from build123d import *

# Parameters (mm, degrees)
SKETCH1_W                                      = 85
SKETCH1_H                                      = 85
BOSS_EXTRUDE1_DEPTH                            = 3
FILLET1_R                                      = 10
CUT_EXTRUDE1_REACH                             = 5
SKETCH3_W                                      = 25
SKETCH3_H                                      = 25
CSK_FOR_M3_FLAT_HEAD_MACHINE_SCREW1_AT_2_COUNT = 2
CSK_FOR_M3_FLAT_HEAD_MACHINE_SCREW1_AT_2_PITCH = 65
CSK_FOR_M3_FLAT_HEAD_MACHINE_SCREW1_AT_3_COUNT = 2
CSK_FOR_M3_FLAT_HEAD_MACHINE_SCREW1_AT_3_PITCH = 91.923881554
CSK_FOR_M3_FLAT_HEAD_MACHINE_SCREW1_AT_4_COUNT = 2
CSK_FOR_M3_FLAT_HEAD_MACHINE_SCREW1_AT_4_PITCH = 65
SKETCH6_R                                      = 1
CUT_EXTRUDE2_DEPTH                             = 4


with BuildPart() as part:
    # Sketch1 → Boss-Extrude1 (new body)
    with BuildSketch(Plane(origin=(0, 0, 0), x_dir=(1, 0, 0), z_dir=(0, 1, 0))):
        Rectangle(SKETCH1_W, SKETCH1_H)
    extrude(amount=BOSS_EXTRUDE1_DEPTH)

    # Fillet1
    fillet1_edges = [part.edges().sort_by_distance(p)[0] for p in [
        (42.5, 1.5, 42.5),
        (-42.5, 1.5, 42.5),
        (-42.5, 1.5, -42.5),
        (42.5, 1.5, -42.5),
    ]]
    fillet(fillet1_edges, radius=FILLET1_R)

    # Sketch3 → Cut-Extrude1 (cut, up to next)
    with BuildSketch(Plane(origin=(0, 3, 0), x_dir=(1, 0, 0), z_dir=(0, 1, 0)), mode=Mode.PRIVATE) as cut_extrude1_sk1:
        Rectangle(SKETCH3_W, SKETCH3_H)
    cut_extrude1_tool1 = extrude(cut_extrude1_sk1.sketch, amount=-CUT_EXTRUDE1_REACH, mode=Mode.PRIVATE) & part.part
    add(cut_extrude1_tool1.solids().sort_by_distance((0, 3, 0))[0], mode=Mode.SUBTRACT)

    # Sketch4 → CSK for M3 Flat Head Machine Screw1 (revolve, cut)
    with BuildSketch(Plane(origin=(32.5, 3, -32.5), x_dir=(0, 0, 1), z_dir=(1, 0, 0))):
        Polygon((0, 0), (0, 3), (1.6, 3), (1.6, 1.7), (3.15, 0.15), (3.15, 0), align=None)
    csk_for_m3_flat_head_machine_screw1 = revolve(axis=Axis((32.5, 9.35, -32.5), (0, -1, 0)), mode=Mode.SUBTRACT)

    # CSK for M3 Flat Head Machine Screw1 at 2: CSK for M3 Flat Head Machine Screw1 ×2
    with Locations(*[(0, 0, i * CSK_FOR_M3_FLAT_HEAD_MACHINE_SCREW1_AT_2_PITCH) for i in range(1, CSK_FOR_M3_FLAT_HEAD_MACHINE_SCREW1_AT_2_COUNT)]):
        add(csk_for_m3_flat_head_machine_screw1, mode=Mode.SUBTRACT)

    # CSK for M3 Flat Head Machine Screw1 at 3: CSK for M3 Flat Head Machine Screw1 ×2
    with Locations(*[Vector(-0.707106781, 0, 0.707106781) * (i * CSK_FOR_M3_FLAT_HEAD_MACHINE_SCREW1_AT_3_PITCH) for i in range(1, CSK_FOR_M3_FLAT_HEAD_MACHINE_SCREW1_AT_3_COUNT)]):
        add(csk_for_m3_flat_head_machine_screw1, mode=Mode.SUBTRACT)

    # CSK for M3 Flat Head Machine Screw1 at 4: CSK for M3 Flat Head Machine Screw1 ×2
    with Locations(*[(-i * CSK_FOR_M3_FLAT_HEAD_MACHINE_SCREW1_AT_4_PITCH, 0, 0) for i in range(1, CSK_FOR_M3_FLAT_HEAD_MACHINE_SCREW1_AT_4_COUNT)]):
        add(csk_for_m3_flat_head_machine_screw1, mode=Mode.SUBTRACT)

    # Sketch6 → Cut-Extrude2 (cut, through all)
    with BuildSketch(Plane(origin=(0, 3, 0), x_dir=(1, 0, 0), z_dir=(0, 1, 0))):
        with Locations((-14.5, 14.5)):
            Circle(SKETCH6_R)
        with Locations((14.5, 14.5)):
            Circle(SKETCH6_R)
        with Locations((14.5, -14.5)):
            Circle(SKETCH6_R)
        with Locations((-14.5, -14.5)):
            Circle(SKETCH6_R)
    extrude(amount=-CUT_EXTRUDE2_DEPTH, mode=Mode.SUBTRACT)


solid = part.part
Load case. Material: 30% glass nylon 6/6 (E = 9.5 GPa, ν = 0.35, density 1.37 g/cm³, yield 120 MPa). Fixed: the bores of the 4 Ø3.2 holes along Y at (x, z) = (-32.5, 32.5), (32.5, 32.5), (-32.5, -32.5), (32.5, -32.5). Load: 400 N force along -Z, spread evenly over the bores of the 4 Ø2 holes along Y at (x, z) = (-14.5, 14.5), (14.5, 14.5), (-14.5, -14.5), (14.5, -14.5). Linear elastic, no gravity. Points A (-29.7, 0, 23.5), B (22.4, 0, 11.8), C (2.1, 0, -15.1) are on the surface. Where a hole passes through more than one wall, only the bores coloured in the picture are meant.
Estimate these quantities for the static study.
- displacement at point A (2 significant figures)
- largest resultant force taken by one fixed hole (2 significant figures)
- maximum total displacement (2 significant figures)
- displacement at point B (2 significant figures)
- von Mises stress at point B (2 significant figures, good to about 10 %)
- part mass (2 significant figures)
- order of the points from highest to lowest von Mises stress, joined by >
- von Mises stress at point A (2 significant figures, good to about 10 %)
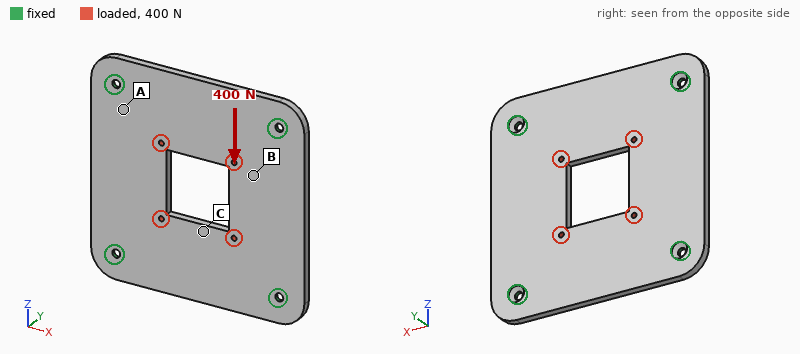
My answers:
4.8 µm
110 N
11 µm
7.2 µm
1.5 MPa
26 g
A > B > C
2.5 MPa
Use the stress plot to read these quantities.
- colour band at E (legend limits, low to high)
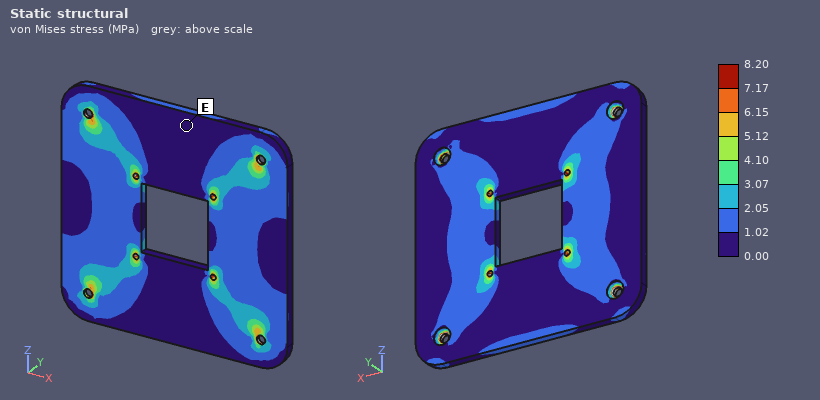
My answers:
0.00 to 1.02 MPa
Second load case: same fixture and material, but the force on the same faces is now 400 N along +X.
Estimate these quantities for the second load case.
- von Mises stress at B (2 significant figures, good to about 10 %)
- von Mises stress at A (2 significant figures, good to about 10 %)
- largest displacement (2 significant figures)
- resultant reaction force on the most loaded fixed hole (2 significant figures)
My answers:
1.2 MPa
2.1 MPa
11 µm
110 N
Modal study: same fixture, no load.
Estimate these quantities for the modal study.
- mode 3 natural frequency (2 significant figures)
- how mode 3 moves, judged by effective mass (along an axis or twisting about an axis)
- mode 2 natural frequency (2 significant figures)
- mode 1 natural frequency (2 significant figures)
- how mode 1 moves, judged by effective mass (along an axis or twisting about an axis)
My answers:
1700 Hz
twisting about Z
1600 Hz
1100 Hz
along Y
